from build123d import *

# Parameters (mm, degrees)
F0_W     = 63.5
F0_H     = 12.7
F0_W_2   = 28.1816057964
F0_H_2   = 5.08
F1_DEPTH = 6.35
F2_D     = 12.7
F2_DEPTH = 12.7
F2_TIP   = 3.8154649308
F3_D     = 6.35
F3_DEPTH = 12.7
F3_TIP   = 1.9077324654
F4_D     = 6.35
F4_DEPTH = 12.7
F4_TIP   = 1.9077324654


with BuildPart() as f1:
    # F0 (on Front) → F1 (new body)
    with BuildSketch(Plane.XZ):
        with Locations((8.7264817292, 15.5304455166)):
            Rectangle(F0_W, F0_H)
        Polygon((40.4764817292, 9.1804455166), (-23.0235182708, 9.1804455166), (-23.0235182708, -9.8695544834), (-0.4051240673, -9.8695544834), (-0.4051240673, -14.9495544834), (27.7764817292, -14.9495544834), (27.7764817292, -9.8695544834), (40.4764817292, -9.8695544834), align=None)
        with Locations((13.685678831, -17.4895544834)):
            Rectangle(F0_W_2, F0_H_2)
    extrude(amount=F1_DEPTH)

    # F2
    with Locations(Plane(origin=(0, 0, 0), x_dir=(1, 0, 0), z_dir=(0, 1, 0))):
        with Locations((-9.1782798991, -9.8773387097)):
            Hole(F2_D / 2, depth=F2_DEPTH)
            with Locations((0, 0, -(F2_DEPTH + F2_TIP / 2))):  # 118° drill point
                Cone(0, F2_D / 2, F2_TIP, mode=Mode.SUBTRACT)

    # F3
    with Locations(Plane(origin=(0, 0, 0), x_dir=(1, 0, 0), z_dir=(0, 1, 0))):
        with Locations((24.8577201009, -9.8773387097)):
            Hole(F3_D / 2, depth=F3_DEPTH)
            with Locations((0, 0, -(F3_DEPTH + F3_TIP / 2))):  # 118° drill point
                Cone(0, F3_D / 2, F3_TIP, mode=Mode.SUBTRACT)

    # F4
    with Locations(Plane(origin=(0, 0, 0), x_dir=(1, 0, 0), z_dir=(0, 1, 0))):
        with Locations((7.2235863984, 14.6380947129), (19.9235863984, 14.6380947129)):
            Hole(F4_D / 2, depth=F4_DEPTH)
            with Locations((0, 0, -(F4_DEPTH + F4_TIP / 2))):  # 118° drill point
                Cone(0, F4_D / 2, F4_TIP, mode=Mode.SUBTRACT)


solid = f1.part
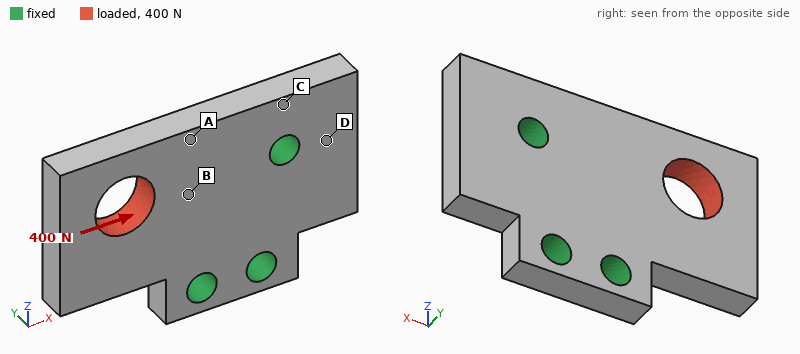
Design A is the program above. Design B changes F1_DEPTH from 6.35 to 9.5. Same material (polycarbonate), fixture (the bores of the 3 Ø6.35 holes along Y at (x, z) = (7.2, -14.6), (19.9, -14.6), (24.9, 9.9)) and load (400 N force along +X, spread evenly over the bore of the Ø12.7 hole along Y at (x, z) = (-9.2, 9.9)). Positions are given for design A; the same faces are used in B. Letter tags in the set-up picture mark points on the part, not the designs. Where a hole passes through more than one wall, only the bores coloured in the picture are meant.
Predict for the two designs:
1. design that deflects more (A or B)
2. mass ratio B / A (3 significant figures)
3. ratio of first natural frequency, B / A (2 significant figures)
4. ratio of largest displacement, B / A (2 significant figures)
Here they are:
A
1.50
1.4
0.67
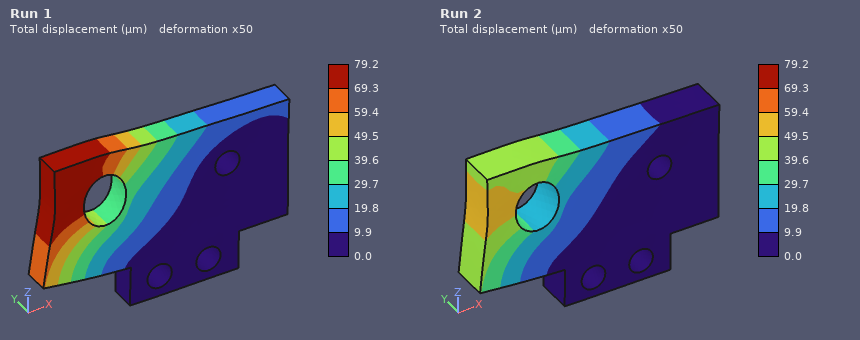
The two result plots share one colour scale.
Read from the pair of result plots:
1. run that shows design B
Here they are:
Run 2
